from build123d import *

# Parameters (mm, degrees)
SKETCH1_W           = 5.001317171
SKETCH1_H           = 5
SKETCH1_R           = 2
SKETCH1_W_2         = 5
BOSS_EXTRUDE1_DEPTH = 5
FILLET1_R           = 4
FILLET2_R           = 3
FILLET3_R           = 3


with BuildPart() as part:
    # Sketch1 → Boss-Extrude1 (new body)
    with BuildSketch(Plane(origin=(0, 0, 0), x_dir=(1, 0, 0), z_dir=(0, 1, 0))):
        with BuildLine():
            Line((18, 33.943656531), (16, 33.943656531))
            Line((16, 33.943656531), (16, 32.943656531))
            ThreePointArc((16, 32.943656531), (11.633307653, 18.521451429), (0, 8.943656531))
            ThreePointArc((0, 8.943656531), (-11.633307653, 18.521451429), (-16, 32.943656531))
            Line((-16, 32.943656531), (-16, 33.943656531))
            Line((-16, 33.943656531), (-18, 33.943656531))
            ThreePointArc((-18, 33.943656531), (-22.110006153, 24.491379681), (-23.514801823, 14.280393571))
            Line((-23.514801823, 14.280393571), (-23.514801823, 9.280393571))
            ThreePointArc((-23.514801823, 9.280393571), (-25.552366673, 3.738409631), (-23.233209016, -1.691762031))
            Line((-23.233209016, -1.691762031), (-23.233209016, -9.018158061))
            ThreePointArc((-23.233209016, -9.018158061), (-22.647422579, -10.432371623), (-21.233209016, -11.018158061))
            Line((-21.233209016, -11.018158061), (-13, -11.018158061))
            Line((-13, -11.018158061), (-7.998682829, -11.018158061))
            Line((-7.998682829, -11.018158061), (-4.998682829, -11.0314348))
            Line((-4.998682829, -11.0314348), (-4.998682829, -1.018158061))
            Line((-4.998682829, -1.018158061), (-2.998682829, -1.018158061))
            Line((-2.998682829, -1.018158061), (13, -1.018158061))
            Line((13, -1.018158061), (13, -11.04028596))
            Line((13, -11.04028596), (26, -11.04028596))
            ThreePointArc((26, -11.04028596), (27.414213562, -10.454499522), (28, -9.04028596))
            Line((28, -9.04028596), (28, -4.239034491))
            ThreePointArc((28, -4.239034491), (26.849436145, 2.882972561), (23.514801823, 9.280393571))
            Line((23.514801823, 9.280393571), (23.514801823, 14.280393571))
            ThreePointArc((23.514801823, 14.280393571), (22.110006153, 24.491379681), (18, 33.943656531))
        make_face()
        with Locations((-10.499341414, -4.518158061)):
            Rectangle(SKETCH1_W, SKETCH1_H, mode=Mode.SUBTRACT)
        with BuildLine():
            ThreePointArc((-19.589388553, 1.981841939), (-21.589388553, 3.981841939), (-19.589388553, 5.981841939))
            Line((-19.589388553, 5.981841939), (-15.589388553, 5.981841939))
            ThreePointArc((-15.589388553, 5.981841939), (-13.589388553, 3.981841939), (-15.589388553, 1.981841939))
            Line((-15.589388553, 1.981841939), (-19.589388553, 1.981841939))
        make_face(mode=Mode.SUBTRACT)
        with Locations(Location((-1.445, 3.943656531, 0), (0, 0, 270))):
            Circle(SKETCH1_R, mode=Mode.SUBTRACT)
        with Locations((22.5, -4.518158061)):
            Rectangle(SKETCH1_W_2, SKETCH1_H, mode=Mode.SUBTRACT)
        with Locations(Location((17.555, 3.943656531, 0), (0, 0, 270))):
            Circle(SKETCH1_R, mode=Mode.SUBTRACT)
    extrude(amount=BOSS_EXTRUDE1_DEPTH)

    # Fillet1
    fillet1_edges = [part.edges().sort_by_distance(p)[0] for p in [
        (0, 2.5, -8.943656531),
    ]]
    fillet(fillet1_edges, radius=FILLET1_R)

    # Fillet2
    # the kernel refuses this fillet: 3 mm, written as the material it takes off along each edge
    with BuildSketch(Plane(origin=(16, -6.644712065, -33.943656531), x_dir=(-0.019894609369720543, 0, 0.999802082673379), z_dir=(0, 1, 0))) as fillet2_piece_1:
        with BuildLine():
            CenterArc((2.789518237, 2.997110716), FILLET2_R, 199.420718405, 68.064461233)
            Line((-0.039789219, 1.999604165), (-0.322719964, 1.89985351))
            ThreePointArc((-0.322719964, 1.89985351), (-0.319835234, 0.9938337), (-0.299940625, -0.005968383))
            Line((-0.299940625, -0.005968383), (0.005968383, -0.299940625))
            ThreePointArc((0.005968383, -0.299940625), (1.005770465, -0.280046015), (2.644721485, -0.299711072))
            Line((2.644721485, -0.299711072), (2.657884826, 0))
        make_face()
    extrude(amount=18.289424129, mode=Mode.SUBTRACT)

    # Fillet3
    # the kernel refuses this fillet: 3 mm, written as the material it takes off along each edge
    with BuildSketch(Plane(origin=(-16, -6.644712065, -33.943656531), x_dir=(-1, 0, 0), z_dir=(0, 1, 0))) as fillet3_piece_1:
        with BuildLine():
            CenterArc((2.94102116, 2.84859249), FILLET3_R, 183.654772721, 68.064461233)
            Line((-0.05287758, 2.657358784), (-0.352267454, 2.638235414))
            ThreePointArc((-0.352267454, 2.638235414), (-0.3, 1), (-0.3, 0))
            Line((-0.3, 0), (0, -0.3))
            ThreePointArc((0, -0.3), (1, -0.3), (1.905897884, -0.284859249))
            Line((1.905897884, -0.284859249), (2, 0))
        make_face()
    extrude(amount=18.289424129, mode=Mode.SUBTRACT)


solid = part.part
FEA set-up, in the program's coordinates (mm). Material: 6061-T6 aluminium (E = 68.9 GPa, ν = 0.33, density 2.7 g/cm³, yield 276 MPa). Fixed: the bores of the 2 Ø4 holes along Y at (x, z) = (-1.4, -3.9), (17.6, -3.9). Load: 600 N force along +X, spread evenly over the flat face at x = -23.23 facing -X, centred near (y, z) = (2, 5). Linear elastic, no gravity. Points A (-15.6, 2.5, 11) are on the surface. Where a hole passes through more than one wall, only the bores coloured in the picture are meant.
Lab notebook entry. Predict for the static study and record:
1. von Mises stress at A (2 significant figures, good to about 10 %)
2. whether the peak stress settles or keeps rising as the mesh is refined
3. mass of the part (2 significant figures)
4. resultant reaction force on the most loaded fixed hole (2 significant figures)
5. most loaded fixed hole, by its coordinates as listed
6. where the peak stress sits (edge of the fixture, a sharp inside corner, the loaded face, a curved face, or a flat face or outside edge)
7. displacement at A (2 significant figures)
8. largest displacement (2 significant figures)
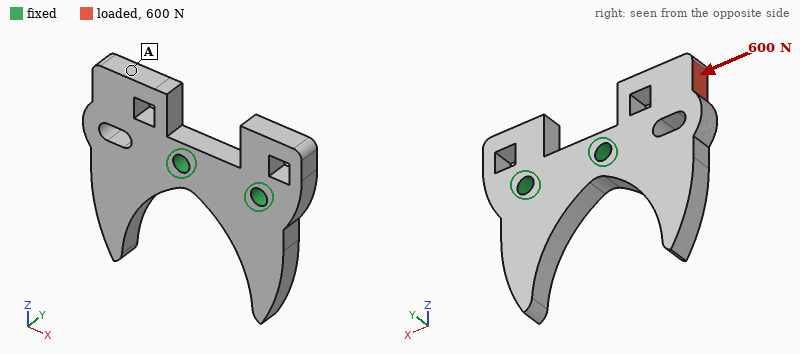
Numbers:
14 MPa
keeps rising
17 g
650 N
(-1.4, -3.9)
edge of the fixture
36 µm
49 µm
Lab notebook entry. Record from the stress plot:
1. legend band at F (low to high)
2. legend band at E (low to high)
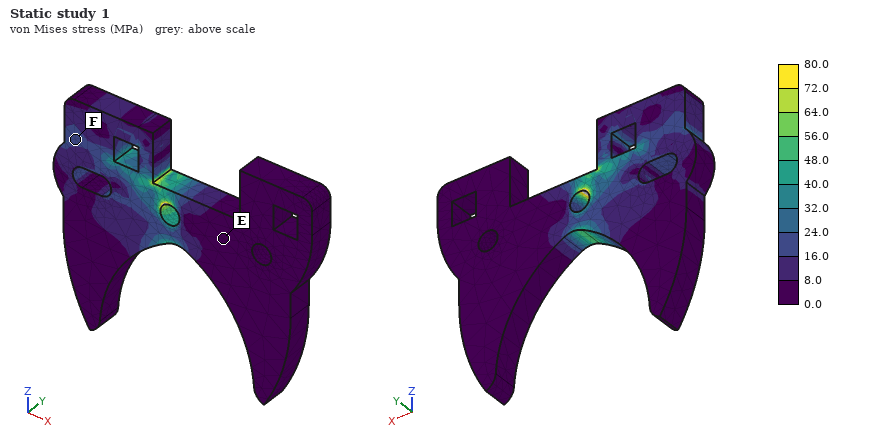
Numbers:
16.0 to 24.0 MPa
0.0 to 8.0 MPa
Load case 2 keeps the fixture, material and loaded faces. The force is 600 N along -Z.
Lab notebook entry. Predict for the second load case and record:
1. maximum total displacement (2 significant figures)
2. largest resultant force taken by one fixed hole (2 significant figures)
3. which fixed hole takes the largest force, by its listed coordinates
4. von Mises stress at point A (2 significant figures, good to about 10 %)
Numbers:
0.11 mm
870 N
(-1.4, -3.9)
19 MPa
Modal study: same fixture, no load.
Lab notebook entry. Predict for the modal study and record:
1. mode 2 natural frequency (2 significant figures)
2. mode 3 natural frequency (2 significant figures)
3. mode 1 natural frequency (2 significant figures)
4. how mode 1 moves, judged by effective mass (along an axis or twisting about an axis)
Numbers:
6100 Hz
6200 Hz
4300 Hz
along Y
